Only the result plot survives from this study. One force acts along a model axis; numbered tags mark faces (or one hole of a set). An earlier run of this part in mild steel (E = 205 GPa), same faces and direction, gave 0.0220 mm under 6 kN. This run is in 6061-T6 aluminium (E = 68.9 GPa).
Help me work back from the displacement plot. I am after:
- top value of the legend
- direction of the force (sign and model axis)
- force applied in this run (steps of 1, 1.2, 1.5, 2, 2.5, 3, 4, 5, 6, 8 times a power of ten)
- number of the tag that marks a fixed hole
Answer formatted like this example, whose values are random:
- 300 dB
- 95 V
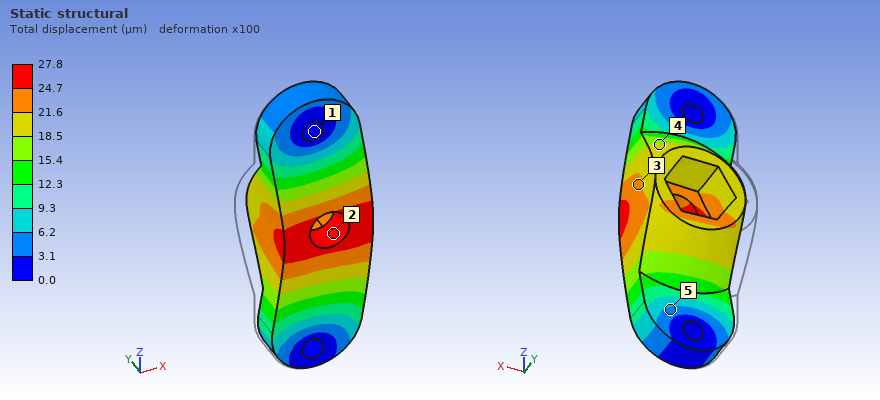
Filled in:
- 27.8 µm
- +X
- 2.5 kN
- 1
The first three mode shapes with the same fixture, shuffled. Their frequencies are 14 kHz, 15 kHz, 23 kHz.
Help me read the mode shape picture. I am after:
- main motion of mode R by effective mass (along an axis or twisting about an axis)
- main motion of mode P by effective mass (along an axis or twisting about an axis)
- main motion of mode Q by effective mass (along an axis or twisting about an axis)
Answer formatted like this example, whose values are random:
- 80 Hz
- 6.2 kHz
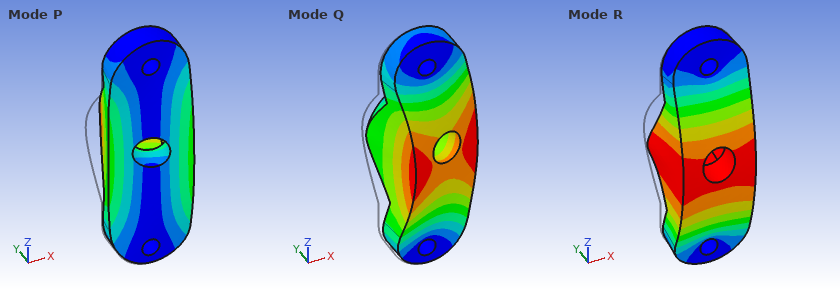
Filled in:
- along Y
- along X
- along X
